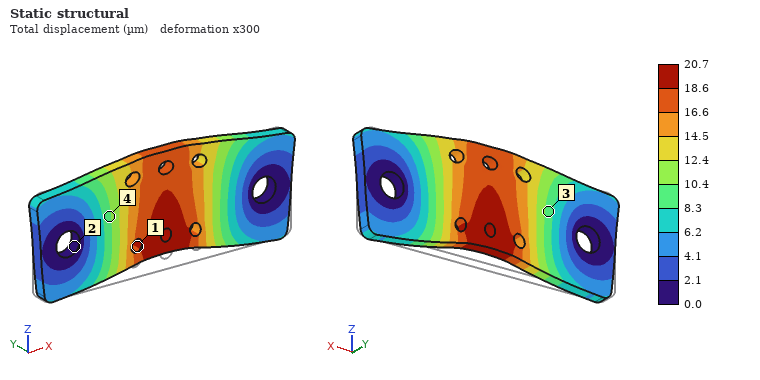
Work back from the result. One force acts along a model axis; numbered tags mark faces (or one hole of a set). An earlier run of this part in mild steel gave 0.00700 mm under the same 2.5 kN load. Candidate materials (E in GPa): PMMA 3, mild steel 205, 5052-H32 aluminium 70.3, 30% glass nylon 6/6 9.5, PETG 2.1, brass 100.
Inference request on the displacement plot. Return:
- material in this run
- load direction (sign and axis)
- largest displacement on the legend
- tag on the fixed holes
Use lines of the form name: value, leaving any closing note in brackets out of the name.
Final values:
material in this run: 5052-H32 aluminium
load direction: +Z
largest displacement on the legend: 20.7 µm
tag on the fixed holes: 2
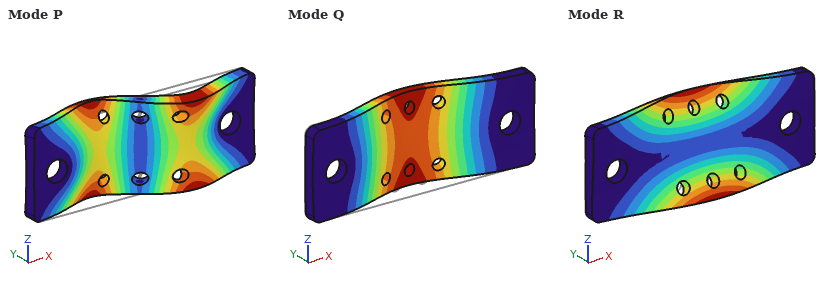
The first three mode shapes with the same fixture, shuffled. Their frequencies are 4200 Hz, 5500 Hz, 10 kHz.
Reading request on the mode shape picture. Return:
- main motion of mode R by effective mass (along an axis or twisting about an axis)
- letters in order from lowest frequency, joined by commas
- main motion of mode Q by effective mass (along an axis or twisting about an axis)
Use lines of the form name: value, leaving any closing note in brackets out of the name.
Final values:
main motion of mode R by effective mass: twisting about X
letters in order from lowest frequency, joined by commas: Q, R, P
main motion of mode Q by effective mass: along Y
